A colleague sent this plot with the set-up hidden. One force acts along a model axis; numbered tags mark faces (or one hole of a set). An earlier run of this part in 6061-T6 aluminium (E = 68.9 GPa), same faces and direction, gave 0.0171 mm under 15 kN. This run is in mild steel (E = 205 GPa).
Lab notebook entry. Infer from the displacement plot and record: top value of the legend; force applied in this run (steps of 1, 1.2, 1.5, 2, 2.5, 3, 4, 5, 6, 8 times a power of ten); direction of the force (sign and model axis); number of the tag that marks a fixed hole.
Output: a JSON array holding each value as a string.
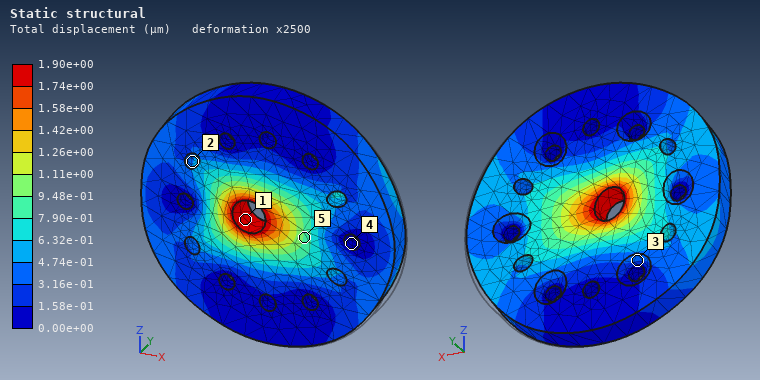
["1.90e+00 µm", "5 kN", "-X", "4"]
